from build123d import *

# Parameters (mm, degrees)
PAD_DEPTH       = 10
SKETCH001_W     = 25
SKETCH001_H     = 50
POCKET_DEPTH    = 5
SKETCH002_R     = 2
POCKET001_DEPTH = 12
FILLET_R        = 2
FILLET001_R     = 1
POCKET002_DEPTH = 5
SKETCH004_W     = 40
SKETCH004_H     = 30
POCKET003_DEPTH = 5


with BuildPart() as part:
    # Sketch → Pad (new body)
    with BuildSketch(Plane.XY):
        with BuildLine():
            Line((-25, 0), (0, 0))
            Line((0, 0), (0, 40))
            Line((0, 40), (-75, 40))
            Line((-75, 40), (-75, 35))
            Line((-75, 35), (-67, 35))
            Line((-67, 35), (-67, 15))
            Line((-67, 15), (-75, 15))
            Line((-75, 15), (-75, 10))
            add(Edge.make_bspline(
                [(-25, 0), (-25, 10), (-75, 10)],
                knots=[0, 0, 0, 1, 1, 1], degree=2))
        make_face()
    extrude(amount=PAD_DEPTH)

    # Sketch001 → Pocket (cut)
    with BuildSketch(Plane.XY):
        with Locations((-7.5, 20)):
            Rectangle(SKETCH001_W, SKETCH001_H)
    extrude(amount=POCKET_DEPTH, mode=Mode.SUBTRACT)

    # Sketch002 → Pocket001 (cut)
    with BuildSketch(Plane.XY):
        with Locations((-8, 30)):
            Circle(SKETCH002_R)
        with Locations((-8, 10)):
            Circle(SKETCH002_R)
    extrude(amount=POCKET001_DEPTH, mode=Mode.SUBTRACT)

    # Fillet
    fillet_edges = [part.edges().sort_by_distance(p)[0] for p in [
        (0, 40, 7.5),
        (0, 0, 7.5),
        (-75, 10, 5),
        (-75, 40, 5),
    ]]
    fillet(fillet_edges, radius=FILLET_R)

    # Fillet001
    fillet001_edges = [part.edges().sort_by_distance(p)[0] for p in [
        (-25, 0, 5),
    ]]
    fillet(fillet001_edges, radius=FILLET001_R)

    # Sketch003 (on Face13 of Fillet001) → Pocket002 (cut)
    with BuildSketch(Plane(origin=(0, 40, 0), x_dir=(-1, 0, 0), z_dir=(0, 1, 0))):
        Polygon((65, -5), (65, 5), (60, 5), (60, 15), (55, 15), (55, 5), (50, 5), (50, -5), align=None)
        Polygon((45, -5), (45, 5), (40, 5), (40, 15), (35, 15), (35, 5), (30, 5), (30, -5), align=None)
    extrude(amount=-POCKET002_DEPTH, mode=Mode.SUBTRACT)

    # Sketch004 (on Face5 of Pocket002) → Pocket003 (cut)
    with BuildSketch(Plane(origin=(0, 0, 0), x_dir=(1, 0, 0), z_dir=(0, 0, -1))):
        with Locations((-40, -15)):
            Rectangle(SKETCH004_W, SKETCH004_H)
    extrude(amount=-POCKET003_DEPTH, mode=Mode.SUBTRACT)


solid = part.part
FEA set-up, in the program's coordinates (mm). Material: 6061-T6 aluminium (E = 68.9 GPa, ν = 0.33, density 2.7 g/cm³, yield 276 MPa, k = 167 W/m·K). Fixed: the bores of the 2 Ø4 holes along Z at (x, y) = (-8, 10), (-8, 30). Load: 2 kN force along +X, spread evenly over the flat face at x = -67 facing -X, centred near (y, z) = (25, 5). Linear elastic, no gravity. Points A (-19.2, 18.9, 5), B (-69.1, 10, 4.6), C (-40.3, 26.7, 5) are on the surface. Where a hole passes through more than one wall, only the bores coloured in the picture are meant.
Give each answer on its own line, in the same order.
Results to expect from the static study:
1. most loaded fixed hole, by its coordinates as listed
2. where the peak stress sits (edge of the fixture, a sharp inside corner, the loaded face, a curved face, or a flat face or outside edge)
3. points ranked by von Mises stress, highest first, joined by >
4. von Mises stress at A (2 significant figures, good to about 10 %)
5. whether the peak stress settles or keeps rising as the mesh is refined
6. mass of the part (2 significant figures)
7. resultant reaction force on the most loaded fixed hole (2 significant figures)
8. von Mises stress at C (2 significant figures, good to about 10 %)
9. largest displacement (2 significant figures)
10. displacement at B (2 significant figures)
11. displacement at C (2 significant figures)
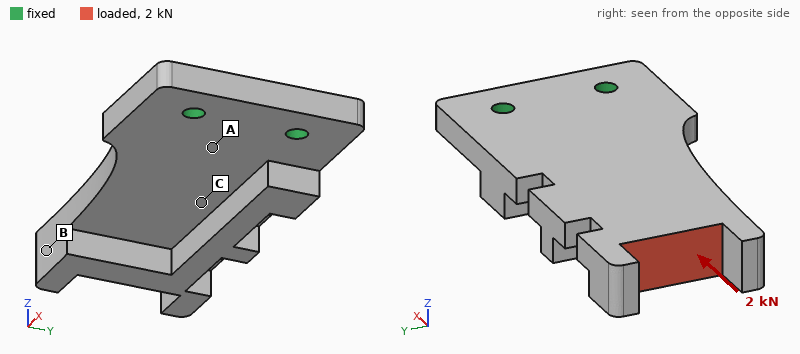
(-8, 30)
edge of the fixture
A > C > B
32 MPa
keeps rising
39 g
1.5 kN
20 MPa
0.27 mm
0.21 mm
0.084 mm
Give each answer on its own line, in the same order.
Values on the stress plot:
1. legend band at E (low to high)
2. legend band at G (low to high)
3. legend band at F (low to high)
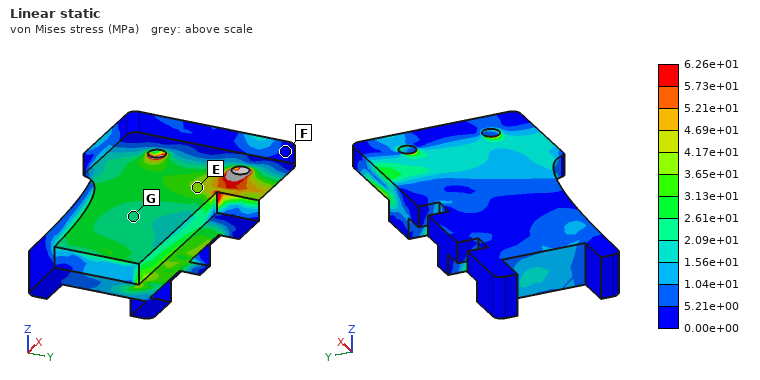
3.65e+01 to 4.17e+01 MPa
2.09e+01 to 2.61e+01 MPa
0.00e+00 to 5.21e+00 MPa
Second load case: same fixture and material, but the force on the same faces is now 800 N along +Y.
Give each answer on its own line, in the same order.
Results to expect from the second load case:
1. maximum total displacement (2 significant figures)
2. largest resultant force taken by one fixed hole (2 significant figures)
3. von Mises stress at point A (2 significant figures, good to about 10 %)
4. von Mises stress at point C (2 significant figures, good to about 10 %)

0.12 mm
2.1 kN
20 MPa
24 MPa
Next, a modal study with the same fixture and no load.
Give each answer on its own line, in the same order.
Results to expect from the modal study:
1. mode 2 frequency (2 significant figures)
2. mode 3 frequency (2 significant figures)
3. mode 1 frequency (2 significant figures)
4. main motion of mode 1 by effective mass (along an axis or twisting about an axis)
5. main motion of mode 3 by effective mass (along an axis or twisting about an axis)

3900 Hz
5000 Hz
1000 Hz
along Z
along Y
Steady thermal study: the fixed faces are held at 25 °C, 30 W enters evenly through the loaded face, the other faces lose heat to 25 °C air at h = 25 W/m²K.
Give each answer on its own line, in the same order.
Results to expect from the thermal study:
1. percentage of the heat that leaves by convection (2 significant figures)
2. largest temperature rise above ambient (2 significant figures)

14 %
55 K
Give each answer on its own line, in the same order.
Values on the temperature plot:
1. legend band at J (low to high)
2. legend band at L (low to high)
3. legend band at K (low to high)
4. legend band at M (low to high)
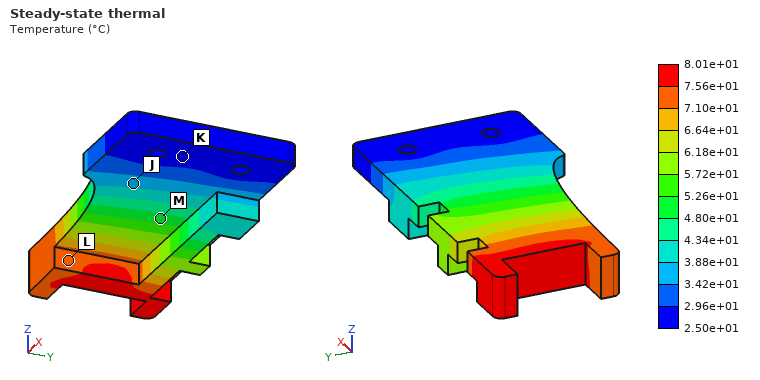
3.42e+01 to 3.88e+01 °C
7.10e+01 to 7.56e+01 °C
2.50e+01 to 2.96e+01 °C
4.80e+01 to 5.26e+01 °C
